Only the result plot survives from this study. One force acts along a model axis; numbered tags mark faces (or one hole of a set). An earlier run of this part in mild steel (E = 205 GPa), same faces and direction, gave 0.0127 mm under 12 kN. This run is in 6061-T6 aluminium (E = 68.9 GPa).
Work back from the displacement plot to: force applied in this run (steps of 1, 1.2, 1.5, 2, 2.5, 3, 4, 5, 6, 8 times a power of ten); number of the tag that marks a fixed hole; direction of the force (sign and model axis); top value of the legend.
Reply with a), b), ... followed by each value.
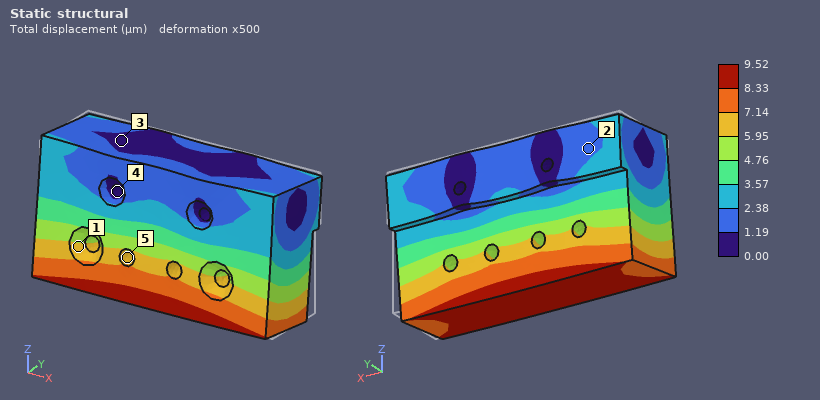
a) 3 kN
b) 4
c) -Y
d) 9.52 µm
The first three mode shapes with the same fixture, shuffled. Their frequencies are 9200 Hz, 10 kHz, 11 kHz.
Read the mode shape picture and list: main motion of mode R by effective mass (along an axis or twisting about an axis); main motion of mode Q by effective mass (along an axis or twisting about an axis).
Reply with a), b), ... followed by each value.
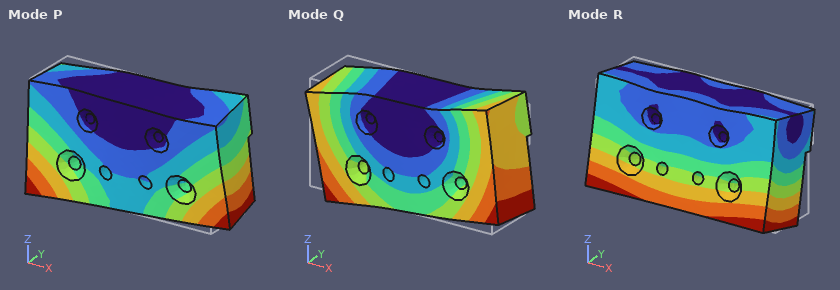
a) along Y
b) along X
